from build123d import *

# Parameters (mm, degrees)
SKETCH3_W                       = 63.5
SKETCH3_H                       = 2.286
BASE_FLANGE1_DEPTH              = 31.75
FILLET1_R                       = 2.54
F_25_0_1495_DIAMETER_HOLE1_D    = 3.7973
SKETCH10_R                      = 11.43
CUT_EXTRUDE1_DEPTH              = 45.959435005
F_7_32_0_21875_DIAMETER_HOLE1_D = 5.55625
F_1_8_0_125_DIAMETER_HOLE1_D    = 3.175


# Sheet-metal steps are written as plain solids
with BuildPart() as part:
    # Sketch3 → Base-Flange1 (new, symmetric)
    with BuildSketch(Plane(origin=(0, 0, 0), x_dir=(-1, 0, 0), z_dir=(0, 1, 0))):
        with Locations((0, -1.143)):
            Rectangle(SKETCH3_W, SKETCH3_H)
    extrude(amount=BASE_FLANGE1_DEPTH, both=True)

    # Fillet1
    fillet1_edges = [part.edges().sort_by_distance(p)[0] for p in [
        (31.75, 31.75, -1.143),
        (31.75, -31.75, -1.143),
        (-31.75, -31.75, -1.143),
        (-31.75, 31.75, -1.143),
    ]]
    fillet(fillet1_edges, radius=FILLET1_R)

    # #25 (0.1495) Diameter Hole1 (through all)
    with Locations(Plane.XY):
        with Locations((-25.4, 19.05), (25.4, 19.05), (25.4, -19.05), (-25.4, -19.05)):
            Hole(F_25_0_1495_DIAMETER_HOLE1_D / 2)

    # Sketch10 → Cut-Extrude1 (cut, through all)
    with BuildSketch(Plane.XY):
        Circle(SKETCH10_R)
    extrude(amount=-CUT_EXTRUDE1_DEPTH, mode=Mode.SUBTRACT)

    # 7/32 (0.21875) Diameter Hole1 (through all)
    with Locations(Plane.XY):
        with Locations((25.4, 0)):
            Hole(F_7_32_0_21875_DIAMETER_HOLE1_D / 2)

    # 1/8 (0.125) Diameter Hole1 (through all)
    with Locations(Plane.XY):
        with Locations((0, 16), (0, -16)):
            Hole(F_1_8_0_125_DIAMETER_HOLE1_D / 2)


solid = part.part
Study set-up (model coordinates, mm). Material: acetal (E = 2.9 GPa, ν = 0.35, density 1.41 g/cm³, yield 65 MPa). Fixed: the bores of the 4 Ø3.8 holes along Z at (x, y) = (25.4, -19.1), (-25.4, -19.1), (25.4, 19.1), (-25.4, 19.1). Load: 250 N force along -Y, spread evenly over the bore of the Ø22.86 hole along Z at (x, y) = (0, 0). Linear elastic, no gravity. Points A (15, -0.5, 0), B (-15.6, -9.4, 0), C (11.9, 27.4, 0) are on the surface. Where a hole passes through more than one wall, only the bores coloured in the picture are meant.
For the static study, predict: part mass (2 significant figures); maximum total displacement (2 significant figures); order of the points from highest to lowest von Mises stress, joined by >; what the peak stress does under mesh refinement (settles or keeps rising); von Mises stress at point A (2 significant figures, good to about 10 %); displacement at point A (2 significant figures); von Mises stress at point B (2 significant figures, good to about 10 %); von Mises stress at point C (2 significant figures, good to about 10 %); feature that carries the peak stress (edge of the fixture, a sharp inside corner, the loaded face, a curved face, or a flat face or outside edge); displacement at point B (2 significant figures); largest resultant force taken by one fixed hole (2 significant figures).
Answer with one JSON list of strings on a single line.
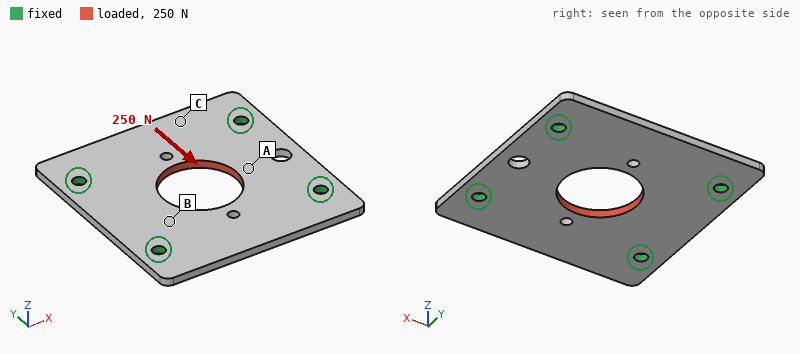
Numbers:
["11 g", "29 µm", "A > B > C", "keeps rising", "2.8 MPa", "15 µm", "1.8 MPa", "1.1 MPa", "edge of the fixture", "13 µm", "66 N"]
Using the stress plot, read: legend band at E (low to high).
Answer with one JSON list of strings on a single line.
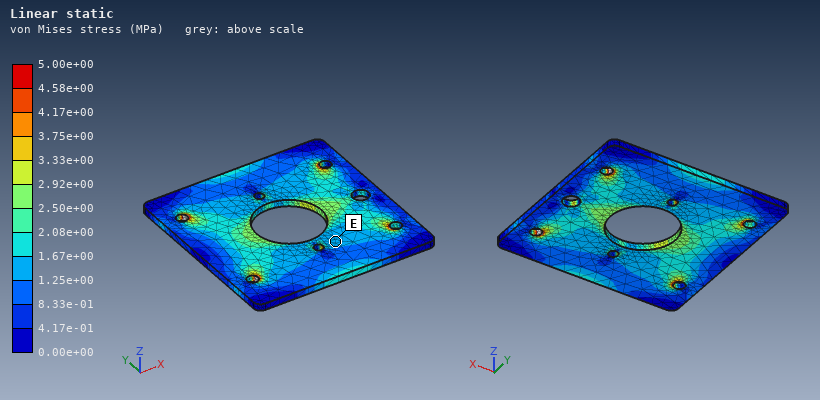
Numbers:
["1.25e+00 to 1.67e+00 MPa"]
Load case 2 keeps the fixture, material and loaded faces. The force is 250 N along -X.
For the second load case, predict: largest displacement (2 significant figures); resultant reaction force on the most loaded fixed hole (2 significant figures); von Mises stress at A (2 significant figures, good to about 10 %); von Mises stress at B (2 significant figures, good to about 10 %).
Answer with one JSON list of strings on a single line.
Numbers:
["19 µm", "67 N", "1.2 MPa", "1.6 MPa"]
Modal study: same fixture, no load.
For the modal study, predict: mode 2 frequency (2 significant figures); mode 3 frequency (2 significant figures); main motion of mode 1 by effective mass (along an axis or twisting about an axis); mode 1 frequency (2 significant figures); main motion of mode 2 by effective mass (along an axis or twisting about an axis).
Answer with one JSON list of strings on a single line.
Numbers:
["1300 Hz", "1600 Hz", "along Z", "1200 Hz", "twisting about X"]
